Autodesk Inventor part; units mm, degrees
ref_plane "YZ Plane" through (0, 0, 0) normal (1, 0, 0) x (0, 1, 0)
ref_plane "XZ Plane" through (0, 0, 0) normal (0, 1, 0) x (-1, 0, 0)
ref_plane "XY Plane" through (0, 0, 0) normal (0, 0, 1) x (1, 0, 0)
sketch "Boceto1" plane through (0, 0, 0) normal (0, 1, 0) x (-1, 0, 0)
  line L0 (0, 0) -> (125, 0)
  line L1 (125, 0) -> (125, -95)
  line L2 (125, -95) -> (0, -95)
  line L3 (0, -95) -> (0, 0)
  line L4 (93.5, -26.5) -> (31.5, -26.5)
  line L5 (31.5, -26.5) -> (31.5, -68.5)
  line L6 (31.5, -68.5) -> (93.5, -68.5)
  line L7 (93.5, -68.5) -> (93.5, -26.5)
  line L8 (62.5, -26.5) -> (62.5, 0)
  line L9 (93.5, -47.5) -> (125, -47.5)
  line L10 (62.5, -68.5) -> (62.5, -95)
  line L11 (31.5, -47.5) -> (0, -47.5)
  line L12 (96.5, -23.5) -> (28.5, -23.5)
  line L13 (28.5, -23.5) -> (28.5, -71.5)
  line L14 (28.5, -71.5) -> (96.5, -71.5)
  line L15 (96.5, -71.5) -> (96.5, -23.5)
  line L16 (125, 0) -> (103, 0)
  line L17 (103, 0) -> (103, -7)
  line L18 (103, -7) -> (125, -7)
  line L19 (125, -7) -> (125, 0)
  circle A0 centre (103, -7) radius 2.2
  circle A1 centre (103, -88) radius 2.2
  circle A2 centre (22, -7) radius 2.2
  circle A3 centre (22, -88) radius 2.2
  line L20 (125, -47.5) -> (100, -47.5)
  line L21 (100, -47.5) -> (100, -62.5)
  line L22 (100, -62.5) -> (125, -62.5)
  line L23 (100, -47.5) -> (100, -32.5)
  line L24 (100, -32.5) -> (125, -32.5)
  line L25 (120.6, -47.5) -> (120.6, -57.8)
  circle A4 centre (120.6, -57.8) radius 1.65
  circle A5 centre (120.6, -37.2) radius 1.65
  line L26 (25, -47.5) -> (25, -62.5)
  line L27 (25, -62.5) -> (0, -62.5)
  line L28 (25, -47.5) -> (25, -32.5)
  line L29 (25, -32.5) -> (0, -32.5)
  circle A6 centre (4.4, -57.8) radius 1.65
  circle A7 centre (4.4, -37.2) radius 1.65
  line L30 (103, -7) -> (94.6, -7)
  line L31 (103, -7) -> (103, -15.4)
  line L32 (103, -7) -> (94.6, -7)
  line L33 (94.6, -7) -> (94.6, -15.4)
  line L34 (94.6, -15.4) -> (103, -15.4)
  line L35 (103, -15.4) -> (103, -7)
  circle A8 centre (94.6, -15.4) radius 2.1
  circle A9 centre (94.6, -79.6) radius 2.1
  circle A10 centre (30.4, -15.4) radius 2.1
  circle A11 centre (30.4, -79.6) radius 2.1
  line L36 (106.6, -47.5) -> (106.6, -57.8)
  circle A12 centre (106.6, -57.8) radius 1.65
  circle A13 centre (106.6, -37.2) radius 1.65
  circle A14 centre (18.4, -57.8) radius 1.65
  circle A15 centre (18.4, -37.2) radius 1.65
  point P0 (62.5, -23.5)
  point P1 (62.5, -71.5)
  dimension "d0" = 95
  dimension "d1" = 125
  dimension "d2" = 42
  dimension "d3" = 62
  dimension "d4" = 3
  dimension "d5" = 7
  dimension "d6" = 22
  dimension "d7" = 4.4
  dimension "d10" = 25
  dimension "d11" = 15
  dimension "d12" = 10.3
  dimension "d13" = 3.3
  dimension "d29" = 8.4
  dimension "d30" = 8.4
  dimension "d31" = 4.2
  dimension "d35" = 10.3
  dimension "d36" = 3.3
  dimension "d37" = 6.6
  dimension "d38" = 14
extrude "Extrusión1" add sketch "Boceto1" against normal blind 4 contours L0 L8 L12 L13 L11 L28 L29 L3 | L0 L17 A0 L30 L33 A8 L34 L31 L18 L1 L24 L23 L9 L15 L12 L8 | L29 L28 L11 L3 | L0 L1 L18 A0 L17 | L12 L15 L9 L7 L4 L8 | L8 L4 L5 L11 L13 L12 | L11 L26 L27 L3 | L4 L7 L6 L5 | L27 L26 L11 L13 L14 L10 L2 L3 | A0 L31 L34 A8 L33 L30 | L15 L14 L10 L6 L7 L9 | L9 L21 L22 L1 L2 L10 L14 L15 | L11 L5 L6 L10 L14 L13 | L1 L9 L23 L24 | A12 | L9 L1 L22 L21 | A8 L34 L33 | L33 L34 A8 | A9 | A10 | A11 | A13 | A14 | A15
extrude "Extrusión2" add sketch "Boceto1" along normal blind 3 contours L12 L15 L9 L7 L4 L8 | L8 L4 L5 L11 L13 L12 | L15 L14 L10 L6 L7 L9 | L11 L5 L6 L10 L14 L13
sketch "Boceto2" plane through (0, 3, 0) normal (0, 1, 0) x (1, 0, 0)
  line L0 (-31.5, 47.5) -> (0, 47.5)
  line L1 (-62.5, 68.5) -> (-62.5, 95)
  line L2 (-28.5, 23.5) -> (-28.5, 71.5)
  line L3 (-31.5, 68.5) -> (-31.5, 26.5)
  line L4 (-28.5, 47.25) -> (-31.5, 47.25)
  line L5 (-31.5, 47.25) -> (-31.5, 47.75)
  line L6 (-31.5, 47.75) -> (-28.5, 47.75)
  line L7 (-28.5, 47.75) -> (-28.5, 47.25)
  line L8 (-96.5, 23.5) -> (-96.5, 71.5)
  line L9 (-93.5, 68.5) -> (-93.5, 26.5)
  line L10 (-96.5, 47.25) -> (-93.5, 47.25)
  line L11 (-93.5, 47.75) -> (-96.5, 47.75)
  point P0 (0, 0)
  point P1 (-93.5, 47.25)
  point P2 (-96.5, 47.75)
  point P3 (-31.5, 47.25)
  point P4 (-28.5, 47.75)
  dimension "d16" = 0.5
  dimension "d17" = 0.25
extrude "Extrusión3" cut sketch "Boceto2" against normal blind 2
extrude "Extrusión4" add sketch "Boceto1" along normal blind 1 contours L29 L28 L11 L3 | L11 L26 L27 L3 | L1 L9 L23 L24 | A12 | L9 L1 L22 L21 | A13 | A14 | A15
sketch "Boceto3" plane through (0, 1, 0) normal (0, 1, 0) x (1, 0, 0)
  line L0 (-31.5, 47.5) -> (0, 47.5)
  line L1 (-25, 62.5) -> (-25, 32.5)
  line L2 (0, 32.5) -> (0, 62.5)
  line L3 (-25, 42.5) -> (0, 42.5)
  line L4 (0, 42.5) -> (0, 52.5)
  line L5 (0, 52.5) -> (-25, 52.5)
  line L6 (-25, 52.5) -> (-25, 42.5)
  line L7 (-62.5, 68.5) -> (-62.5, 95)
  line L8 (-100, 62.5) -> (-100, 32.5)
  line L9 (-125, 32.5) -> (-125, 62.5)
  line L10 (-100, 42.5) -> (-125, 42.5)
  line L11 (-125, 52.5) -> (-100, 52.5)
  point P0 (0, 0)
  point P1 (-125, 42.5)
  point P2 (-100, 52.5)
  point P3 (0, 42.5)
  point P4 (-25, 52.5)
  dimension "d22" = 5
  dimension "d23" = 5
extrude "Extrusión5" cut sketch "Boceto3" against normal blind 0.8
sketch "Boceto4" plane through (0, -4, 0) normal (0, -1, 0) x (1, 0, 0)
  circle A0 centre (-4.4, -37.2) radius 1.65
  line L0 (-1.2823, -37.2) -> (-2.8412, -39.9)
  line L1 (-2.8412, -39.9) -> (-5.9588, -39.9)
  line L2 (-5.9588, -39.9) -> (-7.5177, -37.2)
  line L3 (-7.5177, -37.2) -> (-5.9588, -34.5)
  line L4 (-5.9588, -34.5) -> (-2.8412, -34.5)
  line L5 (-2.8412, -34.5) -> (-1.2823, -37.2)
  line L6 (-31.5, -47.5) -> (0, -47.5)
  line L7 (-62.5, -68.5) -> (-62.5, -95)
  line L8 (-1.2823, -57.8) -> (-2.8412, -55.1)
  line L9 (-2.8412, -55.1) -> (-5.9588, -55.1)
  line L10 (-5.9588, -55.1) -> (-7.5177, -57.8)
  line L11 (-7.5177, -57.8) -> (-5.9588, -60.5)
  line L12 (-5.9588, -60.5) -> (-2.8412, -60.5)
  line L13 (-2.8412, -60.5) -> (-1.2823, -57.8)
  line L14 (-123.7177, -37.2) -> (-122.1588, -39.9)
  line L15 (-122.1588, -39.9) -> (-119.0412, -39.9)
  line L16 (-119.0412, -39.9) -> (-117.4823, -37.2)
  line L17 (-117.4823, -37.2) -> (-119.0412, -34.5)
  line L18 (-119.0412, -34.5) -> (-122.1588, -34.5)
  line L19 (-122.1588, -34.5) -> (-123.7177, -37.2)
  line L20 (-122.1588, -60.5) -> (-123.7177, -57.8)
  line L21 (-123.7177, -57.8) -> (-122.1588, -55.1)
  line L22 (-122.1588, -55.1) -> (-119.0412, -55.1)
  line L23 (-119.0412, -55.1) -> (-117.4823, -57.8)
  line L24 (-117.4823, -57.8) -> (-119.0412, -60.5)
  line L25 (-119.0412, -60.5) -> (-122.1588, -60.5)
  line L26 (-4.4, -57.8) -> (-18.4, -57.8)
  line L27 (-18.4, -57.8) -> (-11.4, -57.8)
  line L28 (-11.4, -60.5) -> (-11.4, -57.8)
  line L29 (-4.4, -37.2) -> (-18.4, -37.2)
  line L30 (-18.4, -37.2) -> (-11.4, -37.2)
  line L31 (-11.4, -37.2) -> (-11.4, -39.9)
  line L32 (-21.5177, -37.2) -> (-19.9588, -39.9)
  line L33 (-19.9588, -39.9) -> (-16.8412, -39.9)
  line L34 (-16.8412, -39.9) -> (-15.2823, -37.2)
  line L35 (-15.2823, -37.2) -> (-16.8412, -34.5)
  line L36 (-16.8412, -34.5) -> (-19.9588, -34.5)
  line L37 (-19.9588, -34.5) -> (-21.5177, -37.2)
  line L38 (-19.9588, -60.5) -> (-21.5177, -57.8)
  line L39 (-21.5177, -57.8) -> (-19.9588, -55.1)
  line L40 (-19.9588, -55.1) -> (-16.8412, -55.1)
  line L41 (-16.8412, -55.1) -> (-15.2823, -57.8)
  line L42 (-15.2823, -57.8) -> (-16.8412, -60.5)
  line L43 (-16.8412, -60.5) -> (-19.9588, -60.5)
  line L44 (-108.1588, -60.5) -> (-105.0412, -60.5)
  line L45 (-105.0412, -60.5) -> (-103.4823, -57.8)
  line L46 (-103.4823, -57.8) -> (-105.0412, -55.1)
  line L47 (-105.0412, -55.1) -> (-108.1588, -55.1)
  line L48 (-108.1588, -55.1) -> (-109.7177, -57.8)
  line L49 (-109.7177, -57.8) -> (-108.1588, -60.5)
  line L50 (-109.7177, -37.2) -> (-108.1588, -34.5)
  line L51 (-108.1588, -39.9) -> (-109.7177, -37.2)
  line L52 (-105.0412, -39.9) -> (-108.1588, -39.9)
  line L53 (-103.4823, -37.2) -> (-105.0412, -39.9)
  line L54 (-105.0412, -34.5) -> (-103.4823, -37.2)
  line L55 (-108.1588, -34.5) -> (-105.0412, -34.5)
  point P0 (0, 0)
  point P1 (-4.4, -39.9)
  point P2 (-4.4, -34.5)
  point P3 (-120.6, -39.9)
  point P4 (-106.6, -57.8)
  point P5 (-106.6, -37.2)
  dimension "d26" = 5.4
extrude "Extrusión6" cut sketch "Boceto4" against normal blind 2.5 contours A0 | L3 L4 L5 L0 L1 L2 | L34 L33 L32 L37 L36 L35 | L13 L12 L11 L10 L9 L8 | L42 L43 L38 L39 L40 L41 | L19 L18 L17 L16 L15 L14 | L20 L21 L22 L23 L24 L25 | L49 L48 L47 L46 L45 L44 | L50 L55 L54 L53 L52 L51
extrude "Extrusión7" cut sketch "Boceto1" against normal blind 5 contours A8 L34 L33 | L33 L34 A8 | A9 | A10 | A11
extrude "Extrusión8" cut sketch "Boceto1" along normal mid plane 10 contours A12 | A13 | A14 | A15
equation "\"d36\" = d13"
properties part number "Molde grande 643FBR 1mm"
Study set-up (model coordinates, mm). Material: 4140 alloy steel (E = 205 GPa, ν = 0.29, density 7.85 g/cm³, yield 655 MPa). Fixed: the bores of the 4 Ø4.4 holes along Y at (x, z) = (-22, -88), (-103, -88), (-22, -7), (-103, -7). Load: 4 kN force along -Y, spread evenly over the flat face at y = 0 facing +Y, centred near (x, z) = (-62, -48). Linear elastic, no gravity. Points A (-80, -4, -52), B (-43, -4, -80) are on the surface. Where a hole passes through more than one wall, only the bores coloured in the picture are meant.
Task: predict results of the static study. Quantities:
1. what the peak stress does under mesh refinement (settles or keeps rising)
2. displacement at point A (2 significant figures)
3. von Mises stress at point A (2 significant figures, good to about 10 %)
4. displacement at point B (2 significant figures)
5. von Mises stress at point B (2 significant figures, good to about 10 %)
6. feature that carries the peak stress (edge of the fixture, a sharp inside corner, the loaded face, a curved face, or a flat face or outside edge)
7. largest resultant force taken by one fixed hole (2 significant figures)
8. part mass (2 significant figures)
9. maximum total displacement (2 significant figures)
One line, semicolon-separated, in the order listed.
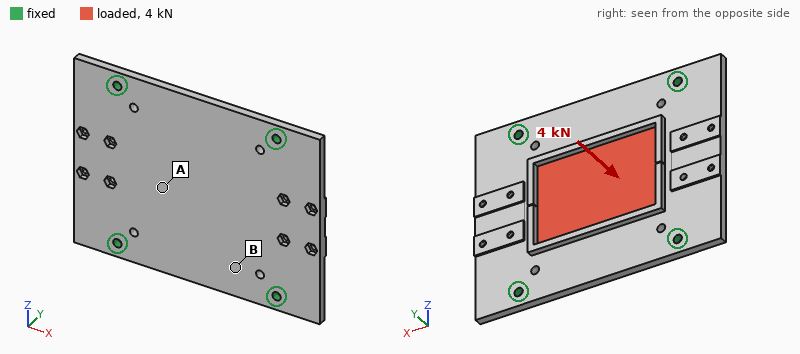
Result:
keeps rising; 0.16 mm; 110 MPa; 0.071 mm; 40 MPa; edge of the fixture; 1.1 kN; 390 g; 0.19 mm
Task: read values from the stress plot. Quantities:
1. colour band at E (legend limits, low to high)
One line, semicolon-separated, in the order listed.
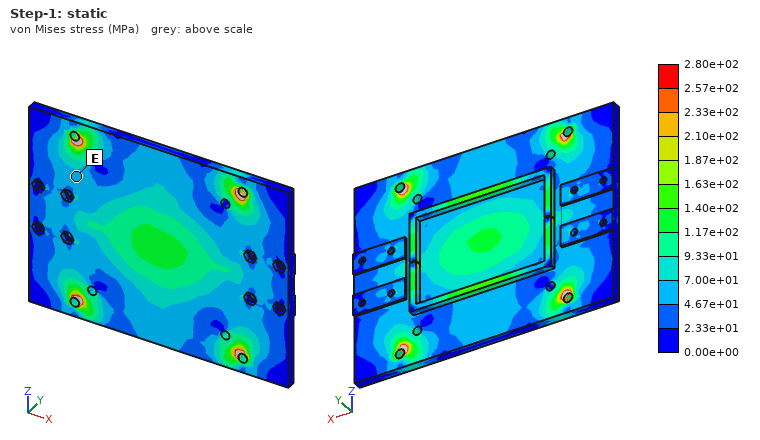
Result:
4.67e+01 to 7.00e+01 MPa
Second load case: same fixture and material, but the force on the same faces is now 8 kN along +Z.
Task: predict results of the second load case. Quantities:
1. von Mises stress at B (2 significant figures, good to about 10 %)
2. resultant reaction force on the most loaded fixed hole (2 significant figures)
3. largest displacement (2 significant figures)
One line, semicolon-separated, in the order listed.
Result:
12 MPa; 2.2 kN; 11 µm
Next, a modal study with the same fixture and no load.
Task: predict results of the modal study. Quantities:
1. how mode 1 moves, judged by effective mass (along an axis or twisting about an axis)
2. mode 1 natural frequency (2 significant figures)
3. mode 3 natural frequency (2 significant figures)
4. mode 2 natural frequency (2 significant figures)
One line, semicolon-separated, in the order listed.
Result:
along Y; 2200 Hz; 3000 Hz; 2900 Hz
